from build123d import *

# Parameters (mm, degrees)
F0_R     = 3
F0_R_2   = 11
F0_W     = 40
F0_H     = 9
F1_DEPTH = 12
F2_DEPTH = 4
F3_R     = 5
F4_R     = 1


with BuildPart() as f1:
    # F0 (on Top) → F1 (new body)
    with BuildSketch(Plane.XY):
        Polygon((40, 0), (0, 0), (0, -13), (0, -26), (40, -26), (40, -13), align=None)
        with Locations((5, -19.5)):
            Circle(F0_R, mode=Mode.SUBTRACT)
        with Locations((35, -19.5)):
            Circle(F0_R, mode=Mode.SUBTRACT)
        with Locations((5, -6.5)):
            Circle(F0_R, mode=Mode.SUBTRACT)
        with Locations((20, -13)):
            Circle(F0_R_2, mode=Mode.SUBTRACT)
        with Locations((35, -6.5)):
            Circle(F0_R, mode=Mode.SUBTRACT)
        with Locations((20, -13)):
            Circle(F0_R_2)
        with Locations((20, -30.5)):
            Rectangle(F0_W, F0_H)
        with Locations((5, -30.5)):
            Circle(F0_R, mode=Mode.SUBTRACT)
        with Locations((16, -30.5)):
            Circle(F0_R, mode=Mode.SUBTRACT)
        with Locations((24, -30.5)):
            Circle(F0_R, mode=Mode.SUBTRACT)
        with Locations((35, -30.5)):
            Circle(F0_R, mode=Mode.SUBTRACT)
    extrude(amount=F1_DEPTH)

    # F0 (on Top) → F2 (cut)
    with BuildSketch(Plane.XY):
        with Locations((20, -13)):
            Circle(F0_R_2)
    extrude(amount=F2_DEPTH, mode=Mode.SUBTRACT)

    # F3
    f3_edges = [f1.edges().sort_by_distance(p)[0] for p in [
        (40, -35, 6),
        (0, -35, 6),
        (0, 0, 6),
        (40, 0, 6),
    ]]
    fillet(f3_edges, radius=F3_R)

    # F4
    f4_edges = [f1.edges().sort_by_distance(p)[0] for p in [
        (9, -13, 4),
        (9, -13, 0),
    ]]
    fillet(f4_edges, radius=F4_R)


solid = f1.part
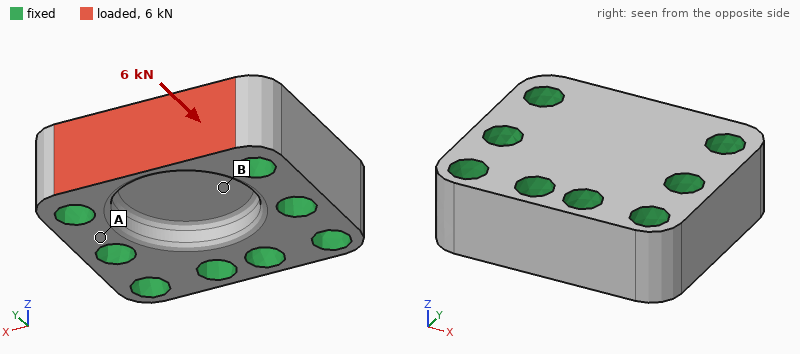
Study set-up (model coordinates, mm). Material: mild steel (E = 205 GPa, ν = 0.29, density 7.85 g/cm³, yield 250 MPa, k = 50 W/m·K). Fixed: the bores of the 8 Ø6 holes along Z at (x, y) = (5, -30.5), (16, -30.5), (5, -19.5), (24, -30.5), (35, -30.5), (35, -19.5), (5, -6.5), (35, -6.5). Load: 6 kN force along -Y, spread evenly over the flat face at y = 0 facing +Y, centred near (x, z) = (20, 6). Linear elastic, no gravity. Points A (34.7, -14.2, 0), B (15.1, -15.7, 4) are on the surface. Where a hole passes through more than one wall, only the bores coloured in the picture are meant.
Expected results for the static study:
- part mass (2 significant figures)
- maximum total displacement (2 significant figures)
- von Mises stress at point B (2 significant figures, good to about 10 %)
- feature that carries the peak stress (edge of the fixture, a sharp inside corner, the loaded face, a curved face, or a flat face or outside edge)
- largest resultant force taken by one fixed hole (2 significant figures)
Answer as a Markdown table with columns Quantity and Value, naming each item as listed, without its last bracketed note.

| Quantity | Value |
|---|---|
| part mass | 97 g |
| maximum total displacement | 6.1 µm |
| von Mises stress at point B | 13 MPa |
| feature that carries the peak stress | a curved face |
| largest resultant force taken by one fixed hole | 2.0 kN |
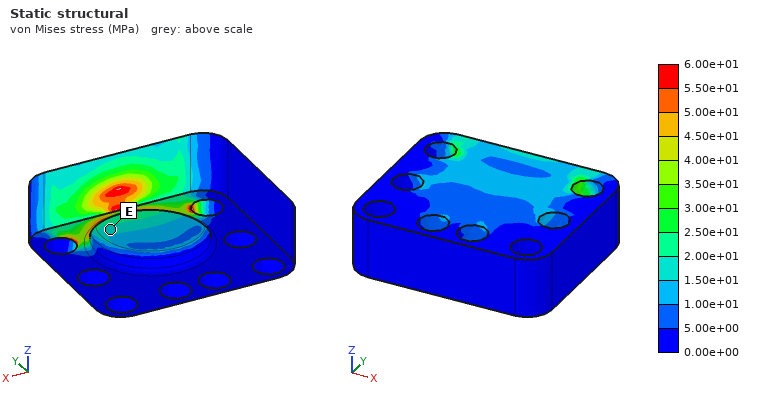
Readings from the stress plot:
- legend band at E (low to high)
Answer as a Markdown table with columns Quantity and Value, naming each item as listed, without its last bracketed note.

| Quantity | Value |
|---|---|
| legend band at E | 1.50e+01 to 2.00e+01 MPa |
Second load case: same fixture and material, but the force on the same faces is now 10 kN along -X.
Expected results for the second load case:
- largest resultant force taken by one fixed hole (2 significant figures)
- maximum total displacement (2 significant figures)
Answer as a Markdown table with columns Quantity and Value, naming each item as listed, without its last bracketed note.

| Quantity | Value |
|---|---|
| largest resultant force taken by one fixed hole | 4.9 kN |
| maximum total displacement | 3.6 µm |
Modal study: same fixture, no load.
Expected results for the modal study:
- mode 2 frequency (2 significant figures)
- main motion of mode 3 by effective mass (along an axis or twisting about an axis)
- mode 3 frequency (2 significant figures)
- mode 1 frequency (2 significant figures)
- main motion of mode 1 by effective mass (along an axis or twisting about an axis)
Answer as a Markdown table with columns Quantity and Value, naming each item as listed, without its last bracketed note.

| Quantity | Value |
|---|---|
| mode 2 frequency | 65 kHz |
| main motion of mode 3 by effective mass | along Y |
| mode 3 frequency | 72 kHz |
| mode 1 frequency | 50 kHz |
| main motion of mode 1 by effective mass | along Z |
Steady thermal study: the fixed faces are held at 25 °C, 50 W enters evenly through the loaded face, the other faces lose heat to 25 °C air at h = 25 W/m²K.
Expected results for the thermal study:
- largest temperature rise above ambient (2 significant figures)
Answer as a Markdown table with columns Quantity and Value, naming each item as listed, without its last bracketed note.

| Quantity | Value |
|---|---|
| largest temperature rise above ambient | 40 K |
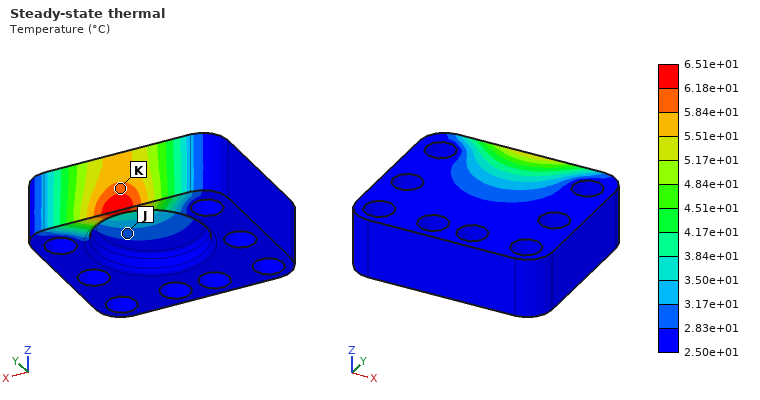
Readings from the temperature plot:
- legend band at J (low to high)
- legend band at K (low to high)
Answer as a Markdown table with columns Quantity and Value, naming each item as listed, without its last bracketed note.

| Quantity | Value |
|---|---|
| legend band at J | 2.83e+01 to 3.17e+01 °C |
| legend band at K | 5.84e+01 to 6.18e+01 °C |
